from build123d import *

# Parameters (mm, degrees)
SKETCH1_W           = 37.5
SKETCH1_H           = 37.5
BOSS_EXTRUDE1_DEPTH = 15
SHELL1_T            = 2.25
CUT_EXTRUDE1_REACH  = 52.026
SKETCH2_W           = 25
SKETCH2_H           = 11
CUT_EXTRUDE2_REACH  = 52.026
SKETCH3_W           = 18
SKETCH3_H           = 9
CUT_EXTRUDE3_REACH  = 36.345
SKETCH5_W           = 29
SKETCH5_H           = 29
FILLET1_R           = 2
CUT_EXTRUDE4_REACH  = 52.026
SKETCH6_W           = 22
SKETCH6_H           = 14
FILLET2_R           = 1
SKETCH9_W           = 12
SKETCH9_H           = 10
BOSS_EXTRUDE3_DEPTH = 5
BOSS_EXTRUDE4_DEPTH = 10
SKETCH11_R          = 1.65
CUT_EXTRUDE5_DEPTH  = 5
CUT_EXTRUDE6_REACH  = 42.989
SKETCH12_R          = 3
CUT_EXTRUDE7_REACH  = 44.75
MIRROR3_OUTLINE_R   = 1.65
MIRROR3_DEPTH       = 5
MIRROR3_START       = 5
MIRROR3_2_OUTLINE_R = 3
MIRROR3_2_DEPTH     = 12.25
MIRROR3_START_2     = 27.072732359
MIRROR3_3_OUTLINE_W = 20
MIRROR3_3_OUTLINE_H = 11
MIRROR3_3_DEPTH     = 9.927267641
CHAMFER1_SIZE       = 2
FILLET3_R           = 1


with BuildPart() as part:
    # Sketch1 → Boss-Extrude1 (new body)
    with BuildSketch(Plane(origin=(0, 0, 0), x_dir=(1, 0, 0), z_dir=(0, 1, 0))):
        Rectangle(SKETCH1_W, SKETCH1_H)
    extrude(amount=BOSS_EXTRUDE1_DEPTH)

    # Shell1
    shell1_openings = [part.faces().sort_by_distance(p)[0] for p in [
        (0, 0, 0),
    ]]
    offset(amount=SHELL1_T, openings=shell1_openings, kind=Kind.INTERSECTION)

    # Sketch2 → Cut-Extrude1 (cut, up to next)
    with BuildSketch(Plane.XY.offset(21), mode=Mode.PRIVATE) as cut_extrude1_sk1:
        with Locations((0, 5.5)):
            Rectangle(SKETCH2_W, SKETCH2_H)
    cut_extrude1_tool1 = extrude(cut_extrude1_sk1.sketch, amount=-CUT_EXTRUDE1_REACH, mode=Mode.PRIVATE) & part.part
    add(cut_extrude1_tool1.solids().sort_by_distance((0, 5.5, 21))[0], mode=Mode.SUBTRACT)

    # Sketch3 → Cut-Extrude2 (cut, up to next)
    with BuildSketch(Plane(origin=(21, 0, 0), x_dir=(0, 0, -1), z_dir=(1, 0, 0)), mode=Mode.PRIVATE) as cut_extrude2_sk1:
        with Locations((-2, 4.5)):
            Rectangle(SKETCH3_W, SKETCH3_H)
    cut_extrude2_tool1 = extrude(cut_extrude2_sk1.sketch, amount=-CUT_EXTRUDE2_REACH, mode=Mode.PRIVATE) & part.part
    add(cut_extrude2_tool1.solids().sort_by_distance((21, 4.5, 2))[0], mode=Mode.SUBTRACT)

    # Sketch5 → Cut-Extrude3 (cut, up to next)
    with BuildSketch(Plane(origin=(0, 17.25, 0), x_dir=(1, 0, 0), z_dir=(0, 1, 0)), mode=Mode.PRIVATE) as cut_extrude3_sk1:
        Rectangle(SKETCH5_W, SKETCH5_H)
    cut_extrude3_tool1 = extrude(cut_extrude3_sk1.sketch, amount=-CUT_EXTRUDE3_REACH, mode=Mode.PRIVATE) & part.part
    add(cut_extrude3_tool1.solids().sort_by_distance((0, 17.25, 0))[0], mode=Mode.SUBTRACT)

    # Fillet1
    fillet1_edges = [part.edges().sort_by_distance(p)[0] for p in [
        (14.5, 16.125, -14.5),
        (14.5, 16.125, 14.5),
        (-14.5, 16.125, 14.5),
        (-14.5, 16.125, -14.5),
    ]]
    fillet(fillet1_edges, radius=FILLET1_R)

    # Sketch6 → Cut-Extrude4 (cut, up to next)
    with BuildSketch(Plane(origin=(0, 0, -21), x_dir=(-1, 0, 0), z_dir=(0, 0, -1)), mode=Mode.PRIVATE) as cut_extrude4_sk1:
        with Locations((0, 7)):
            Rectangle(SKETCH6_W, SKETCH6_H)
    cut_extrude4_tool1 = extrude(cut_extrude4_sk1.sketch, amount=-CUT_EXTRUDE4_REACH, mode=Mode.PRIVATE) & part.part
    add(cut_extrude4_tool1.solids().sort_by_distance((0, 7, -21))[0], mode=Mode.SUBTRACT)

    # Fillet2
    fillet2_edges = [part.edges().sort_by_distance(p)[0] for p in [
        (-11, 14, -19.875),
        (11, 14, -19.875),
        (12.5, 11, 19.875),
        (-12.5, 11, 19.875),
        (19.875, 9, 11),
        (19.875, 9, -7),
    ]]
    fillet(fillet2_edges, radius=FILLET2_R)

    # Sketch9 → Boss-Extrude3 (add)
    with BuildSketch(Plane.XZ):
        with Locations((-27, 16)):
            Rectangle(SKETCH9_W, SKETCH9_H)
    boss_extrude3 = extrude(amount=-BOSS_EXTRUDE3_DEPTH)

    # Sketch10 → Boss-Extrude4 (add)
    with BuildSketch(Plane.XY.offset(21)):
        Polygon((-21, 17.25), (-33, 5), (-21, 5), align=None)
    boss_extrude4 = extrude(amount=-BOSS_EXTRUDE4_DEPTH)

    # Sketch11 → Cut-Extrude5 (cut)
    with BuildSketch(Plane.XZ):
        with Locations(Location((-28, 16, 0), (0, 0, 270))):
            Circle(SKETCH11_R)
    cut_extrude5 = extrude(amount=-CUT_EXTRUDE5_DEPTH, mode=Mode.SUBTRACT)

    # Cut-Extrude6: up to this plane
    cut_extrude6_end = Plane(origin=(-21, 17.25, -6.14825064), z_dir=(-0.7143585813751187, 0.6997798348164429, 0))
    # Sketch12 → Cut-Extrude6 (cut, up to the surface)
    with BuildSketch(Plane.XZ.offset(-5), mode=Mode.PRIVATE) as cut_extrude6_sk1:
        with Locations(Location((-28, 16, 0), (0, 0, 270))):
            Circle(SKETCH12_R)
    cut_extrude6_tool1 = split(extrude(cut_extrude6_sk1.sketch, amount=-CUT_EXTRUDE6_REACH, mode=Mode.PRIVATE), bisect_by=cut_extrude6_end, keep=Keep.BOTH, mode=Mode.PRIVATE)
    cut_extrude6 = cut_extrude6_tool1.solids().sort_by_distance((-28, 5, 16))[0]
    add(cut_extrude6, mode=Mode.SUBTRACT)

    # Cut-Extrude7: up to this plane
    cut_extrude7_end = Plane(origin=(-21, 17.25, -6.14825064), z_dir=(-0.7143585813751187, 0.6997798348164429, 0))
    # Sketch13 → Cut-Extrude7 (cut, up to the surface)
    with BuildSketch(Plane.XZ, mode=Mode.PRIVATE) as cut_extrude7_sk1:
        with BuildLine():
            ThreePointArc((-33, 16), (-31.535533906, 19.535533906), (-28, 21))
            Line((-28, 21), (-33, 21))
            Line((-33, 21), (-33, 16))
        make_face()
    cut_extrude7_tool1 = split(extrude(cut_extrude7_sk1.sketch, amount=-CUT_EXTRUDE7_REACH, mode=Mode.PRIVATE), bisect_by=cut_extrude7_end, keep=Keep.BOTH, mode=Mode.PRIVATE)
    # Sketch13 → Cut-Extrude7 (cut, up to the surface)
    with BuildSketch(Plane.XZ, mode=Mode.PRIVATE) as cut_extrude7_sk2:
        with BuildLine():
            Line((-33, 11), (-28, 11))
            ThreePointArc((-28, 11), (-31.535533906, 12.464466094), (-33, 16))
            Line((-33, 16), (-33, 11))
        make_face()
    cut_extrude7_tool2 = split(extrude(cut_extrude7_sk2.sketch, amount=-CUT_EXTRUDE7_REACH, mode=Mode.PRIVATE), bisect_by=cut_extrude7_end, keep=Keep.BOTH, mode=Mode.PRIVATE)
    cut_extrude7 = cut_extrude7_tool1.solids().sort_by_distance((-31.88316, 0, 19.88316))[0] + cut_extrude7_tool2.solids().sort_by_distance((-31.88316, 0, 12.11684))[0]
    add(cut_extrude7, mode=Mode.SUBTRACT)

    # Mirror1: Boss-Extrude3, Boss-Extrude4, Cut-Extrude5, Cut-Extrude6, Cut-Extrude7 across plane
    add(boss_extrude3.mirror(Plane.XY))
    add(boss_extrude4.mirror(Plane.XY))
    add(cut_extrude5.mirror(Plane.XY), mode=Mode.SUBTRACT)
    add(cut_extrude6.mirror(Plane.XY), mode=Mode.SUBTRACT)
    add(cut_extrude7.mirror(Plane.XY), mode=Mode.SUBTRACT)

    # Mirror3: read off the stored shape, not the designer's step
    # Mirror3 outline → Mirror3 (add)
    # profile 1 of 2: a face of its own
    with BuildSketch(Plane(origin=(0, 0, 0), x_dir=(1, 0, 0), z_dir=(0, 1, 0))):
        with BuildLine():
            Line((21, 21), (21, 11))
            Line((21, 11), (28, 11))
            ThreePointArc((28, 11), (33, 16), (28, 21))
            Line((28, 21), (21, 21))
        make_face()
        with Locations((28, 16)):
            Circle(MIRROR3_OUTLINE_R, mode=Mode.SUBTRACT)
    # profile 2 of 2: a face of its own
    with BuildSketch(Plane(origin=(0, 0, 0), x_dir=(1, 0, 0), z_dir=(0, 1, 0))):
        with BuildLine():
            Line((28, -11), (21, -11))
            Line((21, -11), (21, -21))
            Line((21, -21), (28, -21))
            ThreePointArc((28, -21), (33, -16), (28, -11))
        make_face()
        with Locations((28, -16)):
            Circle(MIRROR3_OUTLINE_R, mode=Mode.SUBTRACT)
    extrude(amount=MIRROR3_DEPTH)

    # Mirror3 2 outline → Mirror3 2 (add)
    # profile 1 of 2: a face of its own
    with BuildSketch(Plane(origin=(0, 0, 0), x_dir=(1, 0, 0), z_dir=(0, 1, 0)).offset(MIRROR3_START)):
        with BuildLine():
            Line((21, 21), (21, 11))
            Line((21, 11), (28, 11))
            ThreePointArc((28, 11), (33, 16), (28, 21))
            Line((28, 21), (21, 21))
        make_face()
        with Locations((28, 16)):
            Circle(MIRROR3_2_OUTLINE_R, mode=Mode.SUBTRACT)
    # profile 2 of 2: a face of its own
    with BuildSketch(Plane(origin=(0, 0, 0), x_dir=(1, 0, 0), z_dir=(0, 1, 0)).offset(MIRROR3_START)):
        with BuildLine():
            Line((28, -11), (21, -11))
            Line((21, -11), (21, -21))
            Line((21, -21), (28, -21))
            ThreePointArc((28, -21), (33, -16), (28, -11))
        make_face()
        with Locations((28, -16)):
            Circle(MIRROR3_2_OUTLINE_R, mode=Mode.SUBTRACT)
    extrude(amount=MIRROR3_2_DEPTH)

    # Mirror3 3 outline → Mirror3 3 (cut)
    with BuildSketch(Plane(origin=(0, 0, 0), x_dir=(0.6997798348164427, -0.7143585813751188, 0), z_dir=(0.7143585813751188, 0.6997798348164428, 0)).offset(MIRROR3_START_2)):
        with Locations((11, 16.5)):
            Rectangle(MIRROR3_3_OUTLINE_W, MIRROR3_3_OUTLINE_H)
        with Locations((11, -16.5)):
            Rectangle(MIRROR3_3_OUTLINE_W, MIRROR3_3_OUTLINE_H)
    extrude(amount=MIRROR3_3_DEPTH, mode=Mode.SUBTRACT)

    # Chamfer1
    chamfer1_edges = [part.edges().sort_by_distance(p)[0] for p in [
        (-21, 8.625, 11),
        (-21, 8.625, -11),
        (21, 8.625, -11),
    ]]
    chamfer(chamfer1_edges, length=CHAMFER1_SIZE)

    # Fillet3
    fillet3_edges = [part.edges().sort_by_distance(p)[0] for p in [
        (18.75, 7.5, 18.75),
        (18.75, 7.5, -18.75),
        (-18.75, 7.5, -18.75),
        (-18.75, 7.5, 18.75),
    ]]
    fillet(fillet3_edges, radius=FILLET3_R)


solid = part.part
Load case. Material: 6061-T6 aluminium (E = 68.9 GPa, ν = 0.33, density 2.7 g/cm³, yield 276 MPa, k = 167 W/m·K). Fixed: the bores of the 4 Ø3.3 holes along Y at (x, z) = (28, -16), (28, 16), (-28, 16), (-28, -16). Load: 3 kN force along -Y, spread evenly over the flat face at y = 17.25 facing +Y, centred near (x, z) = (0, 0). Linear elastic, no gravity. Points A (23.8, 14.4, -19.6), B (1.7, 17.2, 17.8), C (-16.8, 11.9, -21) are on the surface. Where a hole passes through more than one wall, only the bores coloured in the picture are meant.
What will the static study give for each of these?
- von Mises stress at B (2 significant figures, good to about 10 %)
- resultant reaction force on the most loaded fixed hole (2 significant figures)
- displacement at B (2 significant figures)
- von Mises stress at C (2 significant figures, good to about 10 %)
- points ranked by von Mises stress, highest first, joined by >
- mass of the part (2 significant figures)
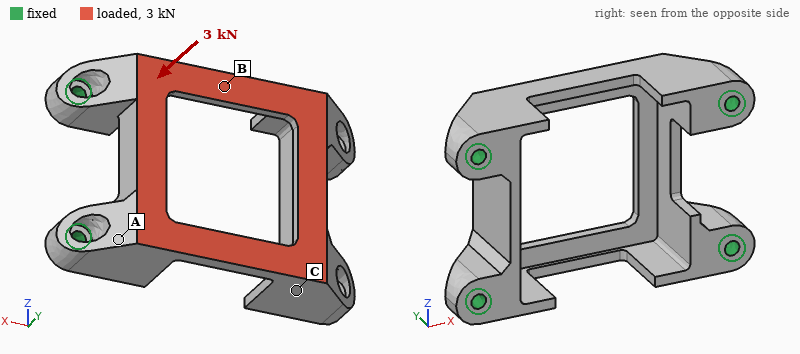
68 MPa
960 N
44 µm
29 MPa
B > C > A
28 g
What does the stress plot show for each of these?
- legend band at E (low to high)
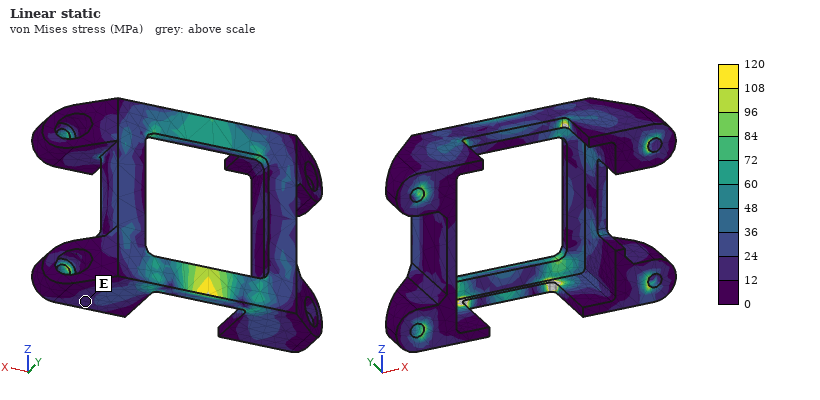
12 to 24 MPa
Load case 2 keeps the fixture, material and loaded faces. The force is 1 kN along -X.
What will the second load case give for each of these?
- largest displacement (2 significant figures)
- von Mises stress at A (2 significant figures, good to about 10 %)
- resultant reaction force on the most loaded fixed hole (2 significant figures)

23 µm
7.3 MPa
270 N
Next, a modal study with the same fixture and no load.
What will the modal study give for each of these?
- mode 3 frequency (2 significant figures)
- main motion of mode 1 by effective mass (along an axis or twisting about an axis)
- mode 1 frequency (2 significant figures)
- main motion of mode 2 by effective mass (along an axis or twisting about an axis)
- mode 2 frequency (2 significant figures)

14 kHz
along X
11 kHz
along Z
12 kHz
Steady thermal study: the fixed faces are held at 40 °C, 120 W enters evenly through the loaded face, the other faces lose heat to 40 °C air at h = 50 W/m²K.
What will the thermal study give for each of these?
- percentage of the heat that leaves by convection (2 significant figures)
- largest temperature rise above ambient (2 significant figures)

6.8 %
68 K
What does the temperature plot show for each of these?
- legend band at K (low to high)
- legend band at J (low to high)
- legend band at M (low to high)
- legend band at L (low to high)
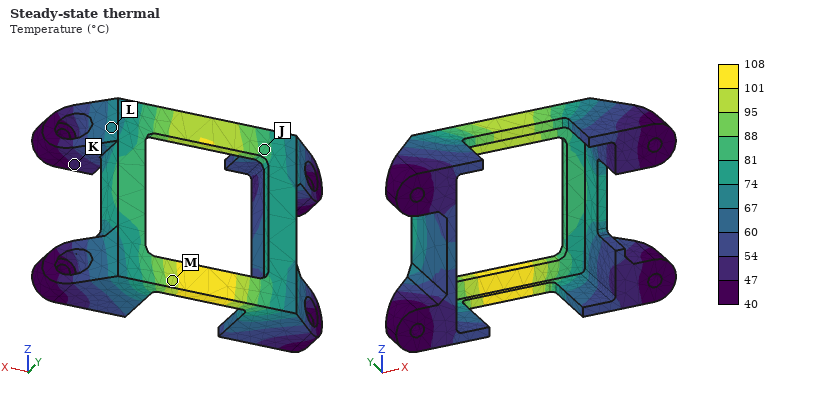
47 to 54 °C
81 to 88 °C
95 to 101 °C
67 to 74 °C
